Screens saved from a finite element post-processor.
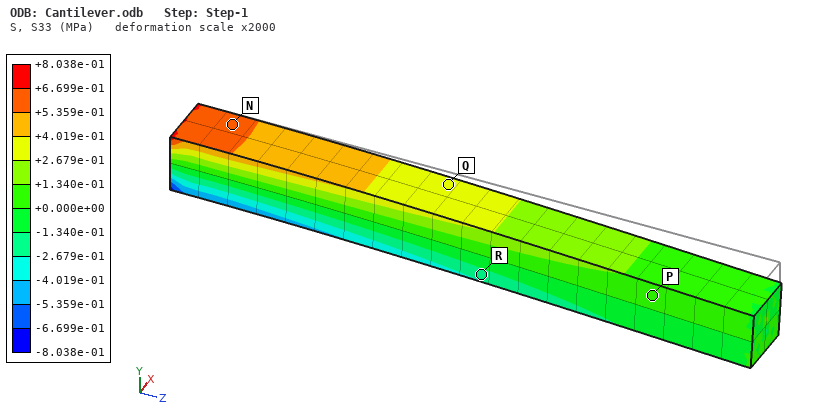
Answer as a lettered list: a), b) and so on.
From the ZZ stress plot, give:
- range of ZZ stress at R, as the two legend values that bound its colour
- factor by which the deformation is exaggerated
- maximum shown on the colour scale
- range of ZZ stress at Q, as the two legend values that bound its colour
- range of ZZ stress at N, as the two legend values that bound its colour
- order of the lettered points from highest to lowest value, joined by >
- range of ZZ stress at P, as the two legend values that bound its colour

a) -2.679e-01 to -1.340e-01 MPa
b) 2000
c) +8.038e-01 MPa
d) +2.679e-01 to +4.019e-01 MPa
e) +5.359e-01 to +6.699e-01 MPa
f) N > Q > P > R
g) +0.000e+00 to +1.340e-01 MPa
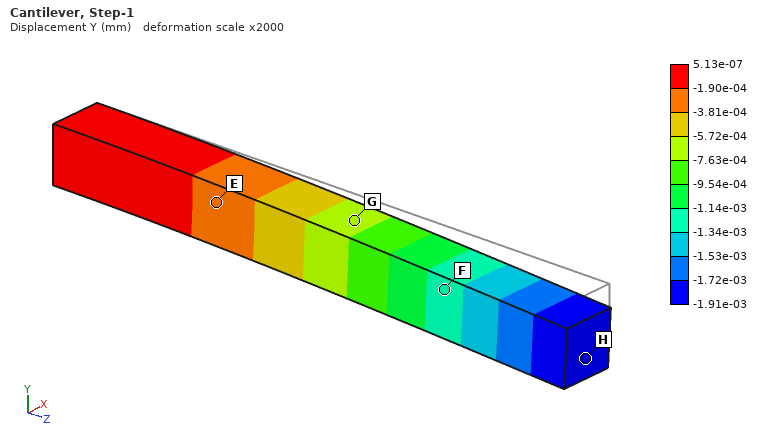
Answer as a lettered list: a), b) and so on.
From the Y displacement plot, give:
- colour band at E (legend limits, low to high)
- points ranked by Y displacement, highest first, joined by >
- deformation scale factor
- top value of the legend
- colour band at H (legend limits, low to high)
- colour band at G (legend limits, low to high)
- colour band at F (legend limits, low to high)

a) -3.81e-04 to -1.90e-04 mm
b) E > G > F > H
c) 2000
d) 5.13e-07 mm
e) -1.91e-03 to -1.72e-03 mm
f) -7.63e-04 to -5.72e-04 mm
g) -1.34e-03 to -1.14e-03 mm
